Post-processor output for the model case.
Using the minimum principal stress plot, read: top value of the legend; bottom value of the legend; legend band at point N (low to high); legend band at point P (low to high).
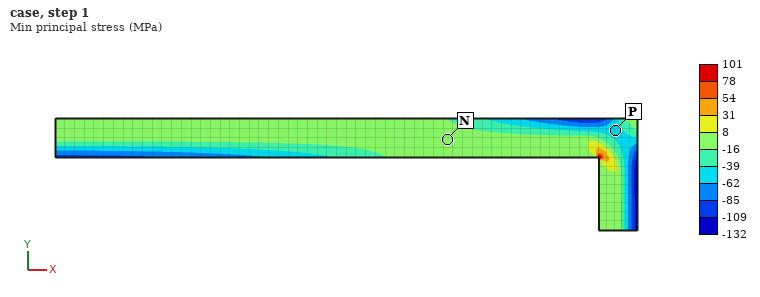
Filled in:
101 MPa
-132 MPa
-16 to 8 MPa
-62 to -39 MPa
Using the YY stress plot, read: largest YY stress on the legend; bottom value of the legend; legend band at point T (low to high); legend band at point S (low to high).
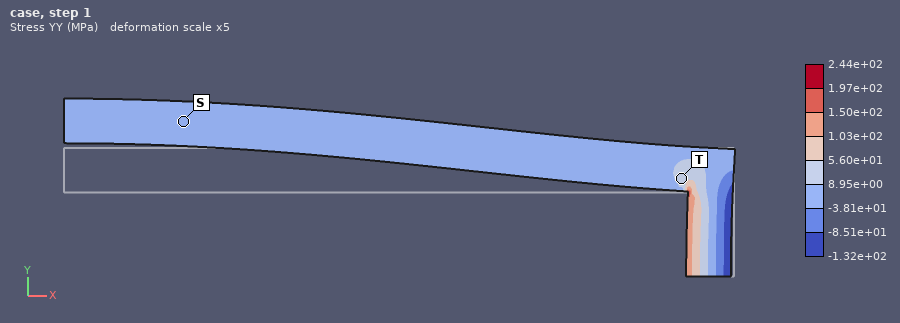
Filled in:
2.44e+02 MPa
-1.32e+02 MPa
8.95e+00 to 5.60e+01 MPa
-3.81e+01 to 8.95e+00 MPa
